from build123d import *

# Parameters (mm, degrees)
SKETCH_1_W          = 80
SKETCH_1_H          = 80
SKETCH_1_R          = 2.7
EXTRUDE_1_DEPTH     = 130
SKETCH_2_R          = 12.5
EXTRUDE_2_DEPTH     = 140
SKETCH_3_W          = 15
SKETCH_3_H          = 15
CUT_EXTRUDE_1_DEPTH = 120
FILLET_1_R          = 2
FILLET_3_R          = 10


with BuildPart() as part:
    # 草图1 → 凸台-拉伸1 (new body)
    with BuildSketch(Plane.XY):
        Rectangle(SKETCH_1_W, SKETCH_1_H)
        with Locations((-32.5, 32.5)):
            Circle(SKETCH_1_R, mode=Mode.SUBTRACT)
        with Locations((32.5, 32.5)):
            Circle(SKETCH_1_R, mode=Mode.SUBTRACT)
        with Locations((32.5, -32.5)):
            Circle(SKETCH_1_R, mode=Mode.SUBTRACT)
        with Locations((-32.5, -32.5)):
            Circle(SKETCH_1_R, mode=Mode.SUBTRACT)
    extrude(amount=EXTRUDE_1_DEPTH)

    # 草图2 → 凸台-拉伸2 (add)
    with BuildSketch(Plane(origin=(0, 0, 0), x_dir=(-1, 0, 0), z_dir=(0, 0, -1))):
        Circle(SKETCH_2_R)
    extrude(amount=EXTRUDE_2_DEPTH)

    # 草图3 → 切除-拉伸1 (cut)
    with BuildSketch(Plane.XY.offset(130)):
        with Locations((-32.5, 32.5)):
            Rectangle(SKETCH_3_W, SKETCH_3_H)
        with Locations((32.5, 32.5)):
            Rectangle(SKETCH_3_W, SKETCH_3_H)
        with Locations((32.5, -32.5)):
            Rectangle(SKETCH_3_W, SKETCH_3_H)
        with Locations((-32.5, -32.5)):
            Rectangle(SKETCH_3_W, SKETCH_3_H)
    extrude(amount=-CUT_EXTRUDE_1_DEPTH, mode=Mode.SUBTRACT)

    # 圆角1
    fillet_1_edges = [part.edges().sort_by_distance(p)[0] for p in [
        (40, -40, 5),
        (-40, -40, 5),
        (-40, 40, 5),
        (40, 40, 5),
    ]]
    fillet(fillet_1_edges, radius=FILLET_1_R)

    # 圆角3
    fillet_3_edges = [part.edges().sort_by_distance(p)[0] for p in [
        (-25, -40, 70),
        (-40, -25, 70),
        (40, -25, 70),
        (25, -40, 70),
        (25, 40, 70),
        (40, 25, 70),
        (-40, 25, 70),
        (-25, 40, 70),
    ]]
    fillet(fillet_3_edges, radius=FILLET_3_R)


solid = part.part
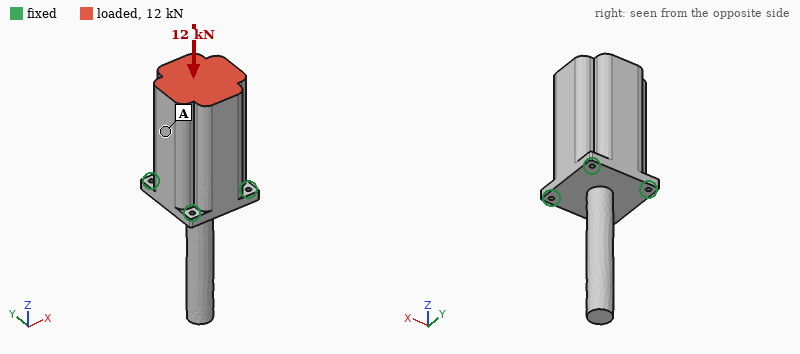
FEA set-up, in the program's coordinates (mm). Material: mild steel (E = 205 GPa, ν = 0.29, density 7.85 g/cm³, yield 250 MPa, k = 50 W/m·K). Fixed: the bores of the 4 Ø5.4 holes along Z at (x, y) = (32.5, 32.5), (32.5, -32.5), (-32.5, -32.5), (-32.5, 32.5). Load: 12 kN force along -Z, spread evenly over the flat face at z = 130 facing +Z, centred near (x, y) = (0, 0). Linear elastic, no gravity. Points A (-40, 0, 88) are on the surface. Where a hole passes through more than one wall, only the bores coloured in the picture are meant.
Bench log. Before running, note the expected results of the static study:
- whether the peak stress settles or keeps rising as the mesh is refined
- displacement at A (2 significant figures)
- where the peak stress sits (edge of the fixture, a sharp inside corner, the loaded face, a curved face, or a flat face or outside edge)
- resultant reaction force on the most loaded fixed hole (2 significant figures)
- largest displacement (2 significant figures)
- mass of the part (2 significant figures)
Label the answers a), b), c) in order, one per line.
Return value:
a) keeps rising
b) 3.9 µm
c) edge of the fixture
d) 3.2 kN
e) 4.4 µm
f) 6.1 kg
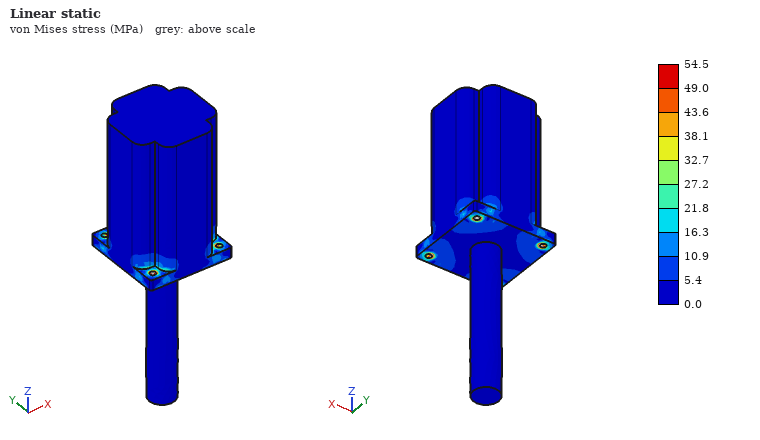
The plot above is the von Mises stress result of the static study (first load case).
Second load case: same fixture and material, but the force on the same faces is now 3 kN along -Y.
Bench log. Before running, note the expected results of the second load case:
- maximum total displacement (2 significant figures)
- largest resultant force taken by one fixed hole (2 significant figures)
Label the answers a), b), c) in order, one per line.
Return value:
a) 18 µm
b) 3.2 kN
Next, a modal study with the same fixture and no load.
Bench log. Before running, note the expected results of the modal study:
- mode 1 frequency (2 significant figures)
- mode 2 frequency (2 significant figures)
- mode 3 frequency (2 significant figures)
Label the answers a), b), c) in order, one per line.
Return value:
a) 810 Hz
b) 810 Hz
c) 1600 Hz
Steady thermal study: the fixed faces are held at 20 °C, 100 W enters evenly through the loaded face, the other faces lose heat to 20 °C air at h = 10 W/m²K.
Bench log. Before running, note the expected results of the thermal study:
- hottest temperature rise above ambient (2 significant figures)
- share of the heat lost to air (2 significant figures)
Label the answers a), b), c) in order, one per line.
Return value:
a) 64 K
b) 18 %
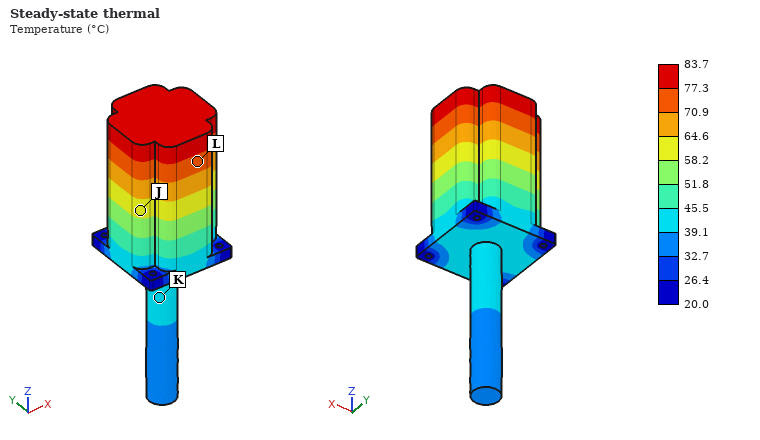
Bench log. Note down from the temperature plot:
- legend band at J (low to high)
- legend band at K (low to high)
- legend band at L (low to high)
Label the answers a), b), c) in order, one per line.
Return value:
a) 58.2 to 64.6 °C
b) 39.1 to 45.5 °C
c) 70.9 to 77.3 °C
